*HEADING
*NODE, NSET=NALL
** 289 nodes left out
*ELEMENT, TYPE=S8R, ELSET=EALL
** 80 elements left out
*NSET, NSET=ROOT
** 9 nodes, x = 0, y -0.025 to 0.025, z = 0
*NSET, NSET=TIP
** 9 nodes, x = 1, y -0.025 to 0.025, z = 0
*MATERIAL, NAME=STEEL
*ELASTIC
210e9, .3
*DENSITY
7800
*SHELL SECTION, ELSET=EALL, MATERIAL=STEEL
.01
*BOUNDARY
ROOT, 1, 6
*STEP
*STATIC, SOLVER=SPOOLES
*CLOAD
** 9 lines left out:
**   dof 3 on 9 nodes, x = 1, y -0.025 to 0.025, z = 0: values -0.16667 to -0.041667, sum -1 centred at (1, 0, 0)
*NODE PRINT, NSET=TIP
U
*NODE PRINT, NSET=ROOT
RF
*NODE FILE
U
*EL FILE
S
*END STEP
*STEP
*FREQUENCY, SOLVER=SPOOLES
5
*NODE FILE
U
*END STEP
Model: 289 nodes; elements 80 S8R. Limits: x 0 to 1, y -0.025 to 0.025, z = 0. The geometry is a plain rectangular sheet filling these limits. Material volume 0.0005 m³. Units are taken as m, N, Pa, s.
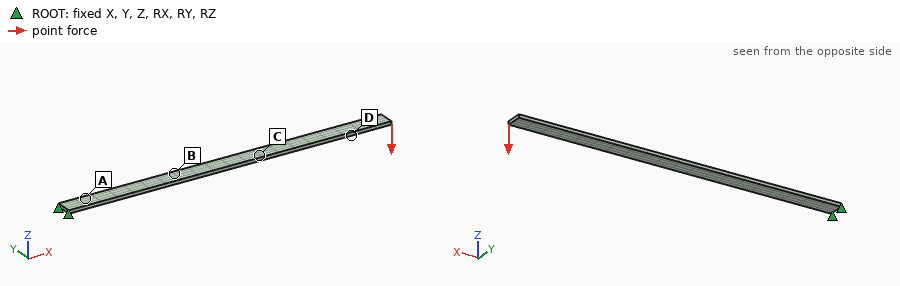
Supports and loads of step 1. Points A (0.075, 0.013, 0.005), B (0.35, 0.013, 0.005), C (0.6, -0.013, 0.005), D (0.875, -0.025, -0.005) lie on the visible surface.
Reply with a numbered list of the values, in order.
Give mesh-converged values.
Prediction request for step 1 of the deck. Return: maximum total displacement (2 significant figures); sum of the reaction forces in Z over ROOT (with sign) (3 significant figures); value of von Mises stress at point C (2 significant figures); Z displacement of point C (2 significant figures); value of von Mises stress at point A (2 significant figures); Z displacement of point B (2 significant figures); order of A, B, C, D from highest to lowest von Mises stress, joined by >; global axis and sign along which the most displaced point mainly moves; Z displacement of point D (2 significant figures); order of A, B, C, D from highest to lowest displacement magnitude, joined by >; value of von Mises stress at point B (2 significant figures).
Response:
1. 3.8e-04 m
2. 1.00 N
3. 4.8e+05 Pa
4. -1.6e-04 m
5. 1.1e+06 Pa
6. -6.1e-05 m
7. A > B > C > D
8. -Z
9. -3.1e-04 m
10. D > C > B > A
11. 7.8e+05 Pa
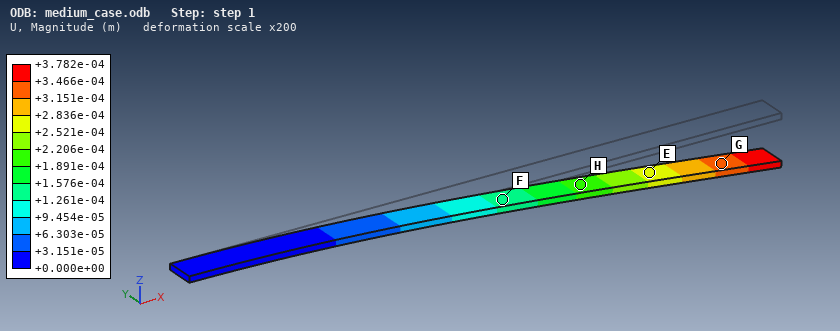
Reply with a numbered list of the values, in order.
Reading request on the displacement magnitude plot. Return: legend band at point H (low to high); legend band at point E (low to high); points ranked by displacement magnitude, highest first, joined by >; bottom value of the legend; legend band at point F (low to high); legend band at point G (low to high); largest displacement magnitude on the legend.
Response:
1. +1.891e-04 to +2.206e-04 m
2. +2.521e-04 to +2.836e-04 m
3. G > E > H > F
4. +0.000e+00 m
5. +1.261e-04 to +1.576e-04 m
6. +3.151e-04 to +3.466e-04 m
7. +3.782e-04 m
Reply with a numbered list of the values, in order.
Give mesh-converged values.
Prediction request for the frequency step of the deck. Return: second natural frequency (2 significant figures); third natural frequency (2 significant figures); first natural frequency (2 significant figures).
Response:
1. 42 Hz
2. 53 Hz
3. 8.4 Hz
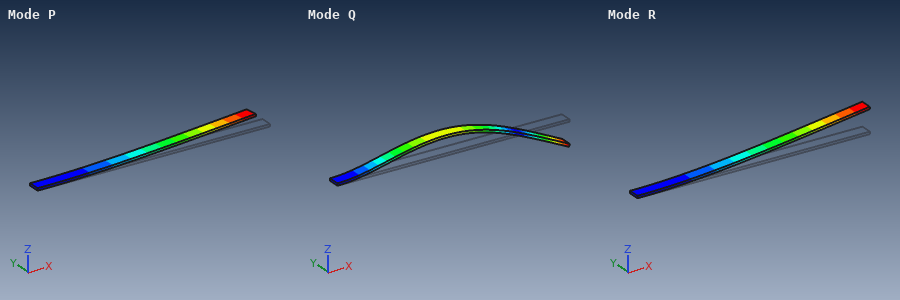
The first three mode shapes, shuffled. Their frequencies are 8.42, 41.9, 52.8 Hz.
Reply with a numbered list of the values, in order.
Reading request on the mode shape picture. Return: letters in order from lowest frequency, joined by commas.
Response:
1. R, P, Q
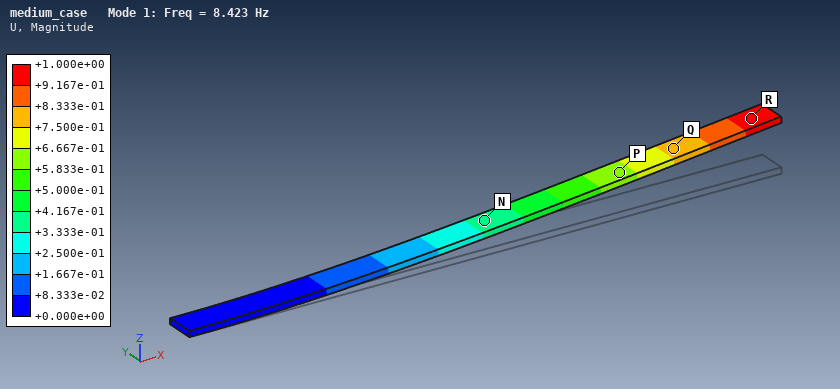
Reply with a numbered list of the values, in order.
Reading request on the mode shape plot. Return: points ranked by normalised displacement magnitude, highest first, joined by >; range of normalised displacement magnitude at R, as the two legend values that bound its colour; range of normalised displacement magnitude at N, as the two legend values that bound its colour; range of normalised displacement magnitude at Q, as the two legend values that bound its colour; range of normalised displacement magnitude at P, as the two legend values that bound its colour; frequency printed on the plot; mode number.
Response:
1. R > Q > P > N
2. +9.167e-01 to +1.000e+00
3. +3.333e-01 to +4.167e-01
4. +7.500e-01 to +8.333e-01
5. +5.833e-01 to +6.667e-01
6. 8.423 Hz
7. 1
